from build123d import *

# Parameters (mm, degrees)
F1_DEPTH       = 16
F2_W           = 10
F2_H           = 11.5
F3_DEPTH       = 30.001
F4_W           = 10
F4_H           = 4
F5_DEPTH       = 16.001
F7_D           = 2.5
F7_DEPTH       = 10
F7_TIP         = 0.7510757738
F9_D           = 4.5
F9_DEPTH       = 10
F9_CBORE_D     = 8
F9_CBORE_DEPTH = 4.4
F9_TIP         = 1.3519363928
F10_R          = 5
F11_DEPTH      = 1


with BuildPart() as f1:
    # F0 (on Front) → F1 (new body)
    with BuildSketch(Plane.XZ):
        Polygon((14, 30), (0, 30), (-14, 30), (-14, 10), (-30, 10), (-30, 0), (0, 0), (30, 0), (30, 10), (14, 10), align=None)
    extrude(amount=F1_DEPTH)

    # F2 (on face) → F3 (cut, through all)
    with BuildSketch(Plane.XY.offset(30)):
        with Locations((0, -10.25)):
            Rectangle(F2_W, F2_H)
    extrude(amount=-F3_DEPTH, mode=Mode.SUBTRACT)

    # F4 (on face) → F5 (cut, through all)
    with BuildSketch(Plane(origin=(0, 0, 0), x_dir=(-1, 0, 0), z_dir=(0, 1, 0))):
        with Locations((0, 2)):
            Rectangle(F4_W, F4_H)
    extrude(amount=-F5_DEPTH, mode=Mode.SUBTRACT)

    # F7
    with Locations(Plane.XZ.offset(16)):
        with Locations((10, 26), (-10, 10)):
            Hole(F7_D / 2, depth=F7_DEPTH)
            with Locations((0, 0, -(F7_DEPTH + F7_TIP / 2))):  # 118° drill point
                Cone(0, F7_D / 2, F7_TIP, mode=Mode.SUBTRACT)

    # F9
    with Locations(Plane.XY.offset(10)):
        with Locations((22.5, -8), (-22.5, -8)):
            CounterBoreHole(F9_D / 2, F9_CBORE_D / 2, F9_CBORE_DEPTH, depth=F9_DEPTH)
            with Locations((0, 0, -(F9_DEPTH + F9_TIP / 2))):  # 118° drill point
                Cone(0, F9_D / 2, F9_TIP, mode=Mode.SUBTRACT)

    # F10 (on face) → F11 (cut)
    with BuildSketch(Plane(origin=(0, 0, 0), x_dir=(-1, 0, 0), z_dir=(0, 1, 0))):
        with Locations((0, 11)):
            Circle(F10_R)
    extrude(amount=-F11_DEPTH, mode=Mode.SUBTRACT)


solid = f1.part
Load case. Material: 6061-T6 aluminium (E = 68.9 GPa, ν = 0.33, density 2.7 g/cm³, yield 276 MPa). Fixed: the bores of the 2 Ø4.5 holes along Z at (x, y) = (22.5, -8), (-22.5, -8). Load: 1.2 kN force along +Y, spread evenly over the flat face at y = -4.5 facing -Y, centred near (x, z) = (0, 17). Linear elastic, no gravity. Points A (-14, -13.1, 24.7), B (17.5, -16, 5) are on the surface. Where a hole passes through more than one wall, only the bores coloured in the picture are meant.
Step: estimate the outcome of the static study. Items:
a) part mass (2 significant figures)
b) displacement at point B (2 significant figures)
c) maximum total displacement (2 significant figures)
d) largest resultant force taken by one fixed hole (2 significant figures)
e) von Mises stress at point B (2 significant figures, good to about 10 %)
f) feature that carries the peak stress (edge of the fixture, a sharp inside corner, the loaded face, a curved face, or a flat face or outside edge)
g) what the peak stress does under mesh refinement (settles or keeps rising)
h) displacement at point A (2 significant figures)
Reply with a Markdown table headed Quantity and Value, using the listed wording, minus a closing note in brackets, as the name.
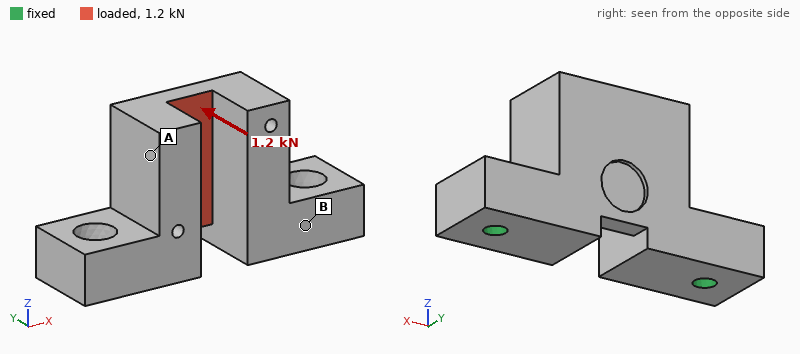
| Quantity | Value |
|---|---|
| part mass | 38 g |
| displacement at point B | 13 µm |
| maximum total displacement | 71 µm |
| largest resultant force taken by one fixed hole | 780 N |
| von Mises stress at point B | 31 MPa |
| feature that carries the peak stress | edge of the fixture |
| what the peak stress does under mesh refinement | keeps rising |
| displacement at point A | 48 µm |
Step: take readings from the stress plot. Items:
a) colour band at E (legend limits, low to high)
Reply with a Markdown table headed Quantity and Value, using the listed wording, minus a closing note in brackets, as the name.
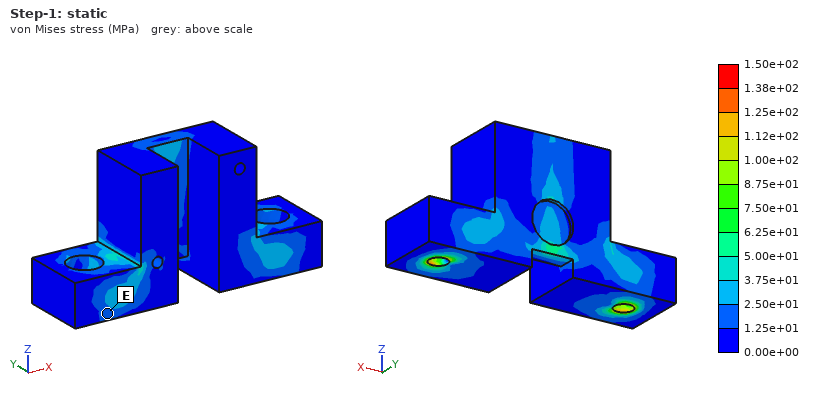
| Quantity | Value |
|---|---|
| colour band at E | 1.25e+01 to 2.50e+01 MPa |
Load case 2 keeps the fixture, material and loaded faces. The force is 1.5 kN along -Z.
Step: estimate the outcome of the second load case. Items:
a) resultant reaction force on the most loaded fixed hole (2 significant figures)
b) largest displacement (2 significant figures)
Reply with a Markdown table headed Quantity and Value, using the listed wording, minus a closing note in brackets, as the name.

| Quantity | Value |
|---|---|
| resultant reaction force on the most loaded fixed hole | 880 N |
| largest displacement | 24 µm |
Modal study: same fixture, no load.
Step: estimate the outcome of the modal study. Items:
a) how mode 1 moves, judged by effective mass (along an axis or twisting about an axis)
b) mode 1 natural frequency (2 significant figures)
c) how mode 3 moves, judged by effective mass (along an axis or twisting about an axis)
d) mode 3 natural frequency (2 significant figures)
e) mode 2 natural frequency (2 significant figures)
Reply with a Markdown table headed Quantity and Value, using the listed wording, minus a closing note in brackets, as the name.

| Quantity | Value |
|---|---|
| how mode 1 moves, judged by effective mass | along Y |
| mode 1 natural frequency | 5400 Hz |
| how mode 3 moves, judged by effective mass | along Z |
| mode 3 natural frequency | 12 kHz |
| mode 2 natural frequency | 10 kHz |
